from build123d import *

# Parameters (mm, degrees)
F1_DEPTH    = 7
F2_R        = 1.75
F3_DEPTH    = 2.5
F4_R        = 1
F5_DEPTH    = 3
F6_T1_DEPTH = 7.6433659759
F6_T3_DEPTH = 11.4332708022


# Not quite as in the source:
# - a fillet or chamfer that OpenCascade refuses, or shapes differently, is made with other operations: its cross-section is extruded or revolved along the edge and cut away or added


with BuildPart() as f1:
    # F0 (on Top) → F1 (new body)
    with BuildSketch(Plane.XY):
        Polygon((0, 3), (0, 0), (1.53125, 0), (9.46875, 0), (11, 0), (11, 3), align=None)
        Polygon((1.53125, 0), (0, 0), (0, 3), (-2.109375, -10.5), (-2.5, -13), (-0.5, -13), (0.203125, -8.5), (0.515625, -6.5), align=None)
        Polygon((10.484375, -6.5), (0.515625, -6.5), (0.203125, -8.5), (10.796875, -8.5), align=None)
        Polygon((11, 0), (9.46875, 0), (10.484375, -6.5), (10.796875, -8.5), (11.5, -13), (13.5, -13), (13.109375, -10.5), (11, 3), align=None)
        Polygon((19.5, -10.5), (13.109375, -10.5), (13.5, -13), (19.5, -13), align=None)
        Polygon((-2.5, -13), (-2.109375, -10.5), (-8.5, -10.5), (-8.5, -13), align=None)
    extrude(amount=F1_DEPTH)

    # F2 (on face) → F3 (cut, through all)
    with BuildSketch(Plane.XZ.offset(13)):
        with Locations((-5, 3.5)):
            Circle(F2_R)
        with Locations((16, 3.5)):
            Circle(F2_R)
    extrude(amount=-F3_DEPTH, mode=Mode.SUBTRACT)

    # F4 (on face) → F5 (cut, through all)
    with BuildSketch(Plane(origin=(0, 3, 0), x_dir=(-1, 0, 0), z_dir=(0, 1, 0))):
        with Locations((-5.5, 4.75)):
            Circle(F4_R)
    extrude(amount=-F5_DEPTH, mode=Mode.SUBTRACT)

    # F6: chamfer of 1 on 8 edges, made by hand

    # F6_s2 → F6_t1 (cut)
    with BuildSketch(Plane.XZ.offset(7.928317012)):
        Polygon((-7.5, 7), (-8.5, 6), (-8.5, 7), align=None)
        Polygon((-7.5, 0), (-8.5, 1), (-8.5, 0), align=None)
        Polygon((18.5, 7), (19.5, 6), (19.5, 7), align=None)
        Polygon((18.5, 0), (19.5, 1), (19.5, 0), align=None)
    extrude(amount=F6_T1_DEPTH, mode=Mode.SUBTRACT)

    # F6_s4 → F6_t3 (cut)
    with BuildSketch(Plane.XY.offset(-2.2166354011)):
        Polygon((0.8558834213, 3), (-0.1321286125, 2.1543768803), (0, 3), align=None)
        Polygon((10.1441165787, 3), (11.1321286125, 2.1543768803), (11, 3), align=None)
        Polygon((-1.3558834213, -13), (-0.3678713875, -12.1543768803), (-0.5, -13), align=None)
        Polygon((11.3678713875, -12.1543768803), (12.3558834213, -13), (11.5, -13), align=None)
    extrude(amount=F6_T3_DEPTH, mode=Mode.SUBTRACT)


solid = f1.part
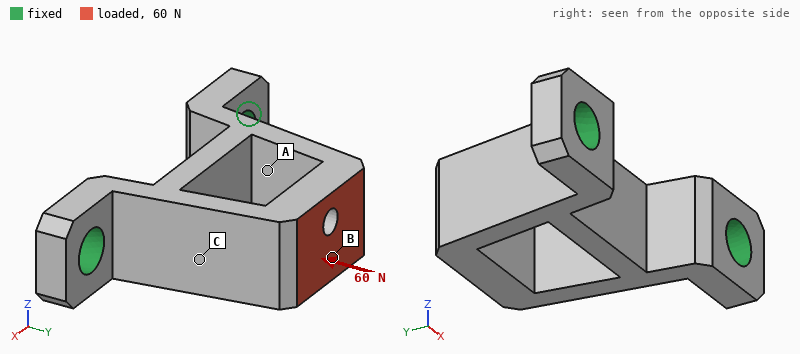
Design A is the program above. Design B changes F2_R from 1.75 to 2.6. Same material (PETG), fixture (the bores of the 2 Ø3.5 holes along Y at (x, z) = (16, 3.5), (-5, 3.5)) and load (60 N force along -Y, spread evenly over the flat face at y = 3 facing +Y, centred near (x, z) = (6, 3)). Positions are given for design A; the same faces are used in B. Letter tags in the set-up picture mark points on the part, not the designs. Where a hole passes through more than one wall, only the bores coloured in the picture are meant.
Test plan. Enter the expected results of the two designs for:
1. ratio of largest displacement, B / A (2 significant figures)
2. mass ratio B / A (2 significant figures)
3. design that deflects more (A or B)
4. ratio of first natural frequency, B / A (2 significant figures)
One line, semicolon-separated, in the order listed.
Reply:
0.86; 0.93; A; 1.2
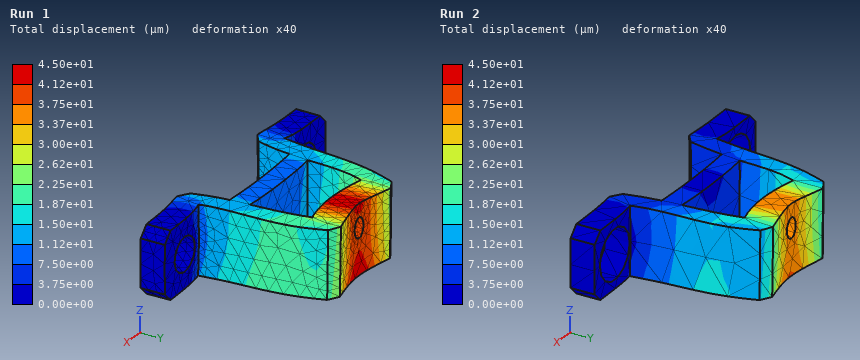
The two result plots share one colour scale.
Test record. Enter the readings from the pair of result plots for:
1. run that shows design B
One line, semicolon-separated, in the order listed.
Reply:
Run 2
